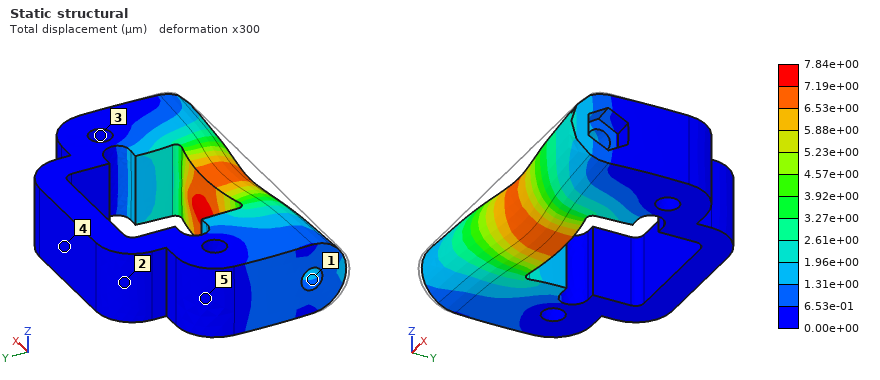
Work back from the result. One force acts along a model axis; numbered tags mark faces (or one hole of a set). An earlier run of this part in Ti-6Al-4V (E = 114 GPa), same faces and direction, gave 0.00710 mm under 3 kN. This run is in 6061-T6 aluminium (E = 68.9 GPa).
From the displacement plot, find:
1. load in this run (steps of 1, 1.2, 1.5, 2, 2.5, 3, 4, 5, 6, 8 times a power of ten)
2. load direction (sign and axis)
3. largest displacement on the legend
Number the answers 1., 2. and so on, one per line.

1. 2 kN
2. +Y
3. 7.84e+00 µm
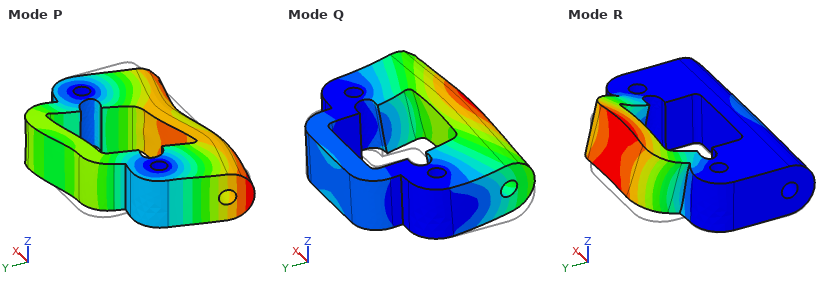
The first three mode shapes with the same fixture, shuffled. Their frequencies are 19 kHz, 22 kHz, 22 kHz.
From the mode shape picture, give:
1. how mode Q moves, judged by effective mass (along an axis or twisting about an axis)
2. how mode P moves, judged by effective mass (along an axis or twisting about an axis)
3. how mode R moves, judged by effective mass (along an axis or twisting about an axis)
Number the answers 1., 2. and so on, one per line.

1. along Z
2. along X
3. along Z
